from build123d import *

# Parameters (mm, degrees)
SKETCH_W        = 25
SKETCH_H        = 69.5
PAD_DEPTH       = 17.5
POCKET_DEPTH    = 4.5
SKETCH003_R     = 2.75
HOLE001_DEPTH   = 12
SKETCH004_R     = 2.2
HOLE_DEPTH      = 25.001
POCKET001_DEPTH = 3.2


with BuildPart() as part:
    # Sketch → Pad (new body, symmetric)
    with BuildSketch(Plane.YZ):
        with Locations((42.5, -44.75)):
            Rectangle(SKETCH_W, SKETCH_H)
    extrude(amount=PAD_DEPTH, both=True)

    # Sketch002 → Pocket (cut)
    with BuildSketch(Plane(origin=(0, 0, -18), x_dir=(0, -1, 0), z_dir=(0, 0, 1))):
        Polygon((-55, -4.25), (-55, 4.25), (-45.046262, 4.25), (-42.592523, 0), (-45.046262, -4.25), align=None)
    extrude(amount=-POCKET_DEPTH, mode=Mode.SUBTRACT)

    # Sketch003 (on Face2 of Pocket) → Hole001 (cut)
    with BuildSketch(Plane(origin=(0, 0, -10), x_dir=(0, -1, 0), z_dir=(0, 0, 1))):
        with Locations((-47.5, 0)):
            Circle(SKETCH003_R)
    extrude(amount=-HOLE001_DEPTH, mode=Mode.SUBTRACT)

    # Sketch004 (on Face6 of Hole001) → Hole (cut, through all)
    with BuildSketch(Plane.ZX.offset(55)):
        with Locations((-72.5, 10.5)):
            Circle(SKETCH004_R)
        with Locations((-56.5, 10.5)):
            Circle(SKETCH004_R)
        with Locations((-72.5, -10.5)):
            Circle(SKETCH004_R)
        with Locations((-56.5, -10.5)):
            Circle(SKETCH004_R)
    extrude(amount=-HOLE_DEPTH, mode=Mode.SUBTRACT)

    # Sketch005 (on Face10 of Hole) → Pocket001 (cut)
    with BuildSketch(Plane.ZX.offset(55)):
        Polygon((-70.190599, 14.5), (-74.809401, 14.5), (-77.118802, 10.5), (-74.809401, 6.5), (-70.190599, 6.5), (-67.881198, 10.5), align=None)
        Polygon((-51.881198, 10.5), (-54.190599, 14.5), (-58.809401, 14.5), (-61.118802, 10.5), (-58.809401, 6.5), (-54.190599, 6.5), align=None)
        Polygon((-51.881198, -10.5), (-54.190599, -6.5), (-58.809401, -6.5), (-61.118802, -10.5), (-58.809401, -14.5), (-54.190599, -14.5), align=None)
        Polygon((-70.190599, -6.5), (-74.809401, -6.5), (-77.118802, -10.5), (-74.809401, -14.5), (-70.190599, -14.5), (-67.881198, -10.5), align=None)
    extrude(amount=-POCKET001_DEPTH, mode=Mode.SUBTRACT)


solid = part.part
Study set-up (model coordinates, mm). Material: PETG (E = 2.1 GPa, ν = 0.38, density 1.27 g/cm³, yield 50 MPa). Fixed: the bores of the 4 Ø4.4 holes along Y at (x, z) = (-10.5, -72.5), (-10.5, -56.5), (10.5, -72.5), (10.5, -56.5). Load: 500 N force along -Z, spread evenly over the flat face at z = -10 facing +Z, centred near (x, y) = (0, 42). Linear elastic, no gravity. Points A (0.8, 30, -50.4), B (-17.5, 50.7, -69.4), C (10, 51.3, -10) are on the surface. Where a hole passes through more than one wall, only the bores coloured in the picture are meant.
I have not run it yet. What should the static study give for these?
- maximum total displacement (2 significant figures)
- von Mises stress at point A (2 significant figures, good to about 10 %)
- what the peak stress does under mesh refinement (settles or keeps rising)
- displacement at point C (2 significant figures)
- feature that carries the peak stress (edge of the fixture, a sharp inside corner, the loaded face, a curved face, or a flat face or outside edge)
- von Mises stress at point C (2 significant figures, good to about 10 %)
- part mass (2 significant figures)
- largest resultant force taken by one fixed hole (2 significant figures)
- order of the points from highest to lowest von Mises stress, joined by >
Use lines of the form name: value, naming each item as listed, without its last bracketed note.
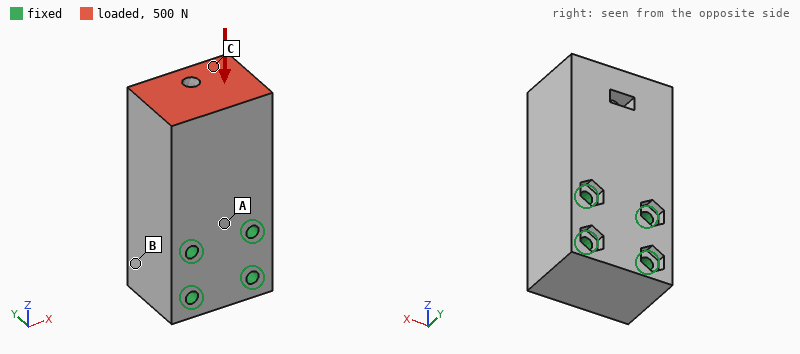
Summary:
maximum total displacement: 18 µm
von Mises stress at point A: 0.29 MPa
what the peak stress does under mesh refinement: keeps rising
displacement at point C: 15 µm
feature that carries the peak stress: edge of the fixture
von Mises stress at point C: 0.65 MPa
part mass: 74 g
largest resultant force taken by one fixed hole: 210 N
order of the points from highest to lowest von Mises stress, joined by >: C > A > B
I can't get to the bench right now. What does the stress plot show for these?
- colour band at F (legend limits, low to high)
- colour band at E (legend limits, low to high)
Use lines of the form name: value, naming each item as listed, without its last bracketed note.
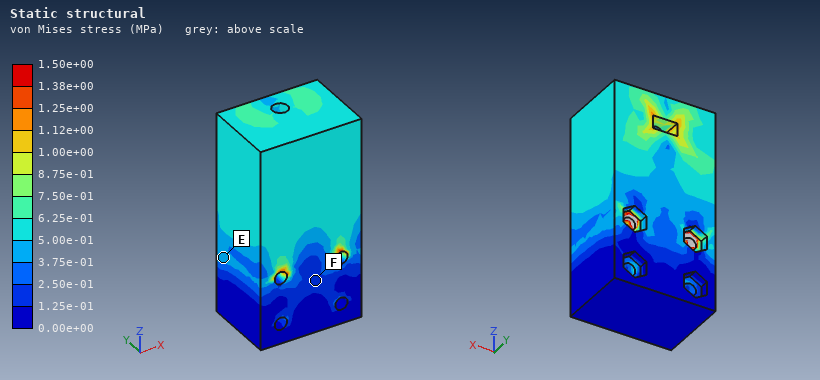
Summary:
colour band at F: 1.25e-01 to 2.50e-01 MPa
colour band at E: 3.75e-01 to 5.00e-01 MPa
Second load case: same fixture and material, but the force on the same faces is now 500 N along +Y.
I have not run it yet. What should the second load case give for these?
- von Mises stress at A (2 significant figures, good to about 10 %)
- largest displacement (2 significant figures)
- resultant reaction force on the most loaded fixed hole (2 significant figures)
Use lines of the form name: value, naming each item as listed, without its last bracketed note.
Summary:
von Mises stress at A: 4.0 MPa
largest displacement: 0.28 mm
resultant reaction force on the most loaded fixed hole: 350 N
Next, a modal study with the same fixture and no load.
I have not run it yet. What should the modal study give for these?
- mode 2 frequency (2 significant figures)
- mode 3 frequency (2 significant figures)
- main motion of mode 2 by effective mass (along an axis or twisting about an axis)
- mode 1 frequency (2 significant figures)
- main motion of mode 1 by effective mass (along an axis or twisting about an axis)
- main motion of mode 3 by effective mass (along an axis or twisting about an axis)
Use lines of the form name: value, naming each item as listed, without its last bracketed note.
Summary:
mode 2 frequency: 2400 Hz
mode 3 frequency: 3700 Hz
main motion of mode 2 by effective mass: along X
mode 1 frequency: 1800 Hz
main motion of mode 1 by effective mass: along Y
main motion of mode 3 by effective mass: twisting about Z
